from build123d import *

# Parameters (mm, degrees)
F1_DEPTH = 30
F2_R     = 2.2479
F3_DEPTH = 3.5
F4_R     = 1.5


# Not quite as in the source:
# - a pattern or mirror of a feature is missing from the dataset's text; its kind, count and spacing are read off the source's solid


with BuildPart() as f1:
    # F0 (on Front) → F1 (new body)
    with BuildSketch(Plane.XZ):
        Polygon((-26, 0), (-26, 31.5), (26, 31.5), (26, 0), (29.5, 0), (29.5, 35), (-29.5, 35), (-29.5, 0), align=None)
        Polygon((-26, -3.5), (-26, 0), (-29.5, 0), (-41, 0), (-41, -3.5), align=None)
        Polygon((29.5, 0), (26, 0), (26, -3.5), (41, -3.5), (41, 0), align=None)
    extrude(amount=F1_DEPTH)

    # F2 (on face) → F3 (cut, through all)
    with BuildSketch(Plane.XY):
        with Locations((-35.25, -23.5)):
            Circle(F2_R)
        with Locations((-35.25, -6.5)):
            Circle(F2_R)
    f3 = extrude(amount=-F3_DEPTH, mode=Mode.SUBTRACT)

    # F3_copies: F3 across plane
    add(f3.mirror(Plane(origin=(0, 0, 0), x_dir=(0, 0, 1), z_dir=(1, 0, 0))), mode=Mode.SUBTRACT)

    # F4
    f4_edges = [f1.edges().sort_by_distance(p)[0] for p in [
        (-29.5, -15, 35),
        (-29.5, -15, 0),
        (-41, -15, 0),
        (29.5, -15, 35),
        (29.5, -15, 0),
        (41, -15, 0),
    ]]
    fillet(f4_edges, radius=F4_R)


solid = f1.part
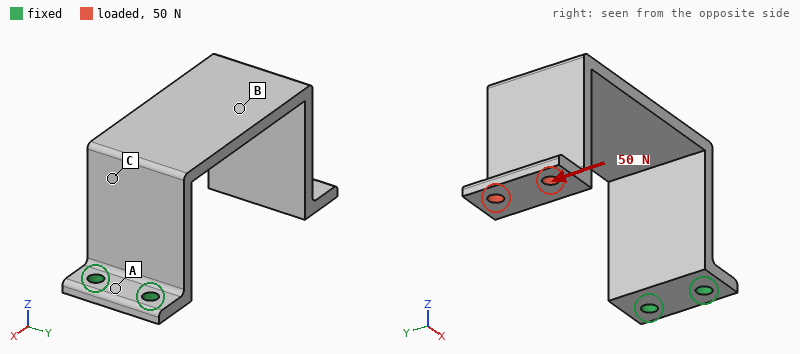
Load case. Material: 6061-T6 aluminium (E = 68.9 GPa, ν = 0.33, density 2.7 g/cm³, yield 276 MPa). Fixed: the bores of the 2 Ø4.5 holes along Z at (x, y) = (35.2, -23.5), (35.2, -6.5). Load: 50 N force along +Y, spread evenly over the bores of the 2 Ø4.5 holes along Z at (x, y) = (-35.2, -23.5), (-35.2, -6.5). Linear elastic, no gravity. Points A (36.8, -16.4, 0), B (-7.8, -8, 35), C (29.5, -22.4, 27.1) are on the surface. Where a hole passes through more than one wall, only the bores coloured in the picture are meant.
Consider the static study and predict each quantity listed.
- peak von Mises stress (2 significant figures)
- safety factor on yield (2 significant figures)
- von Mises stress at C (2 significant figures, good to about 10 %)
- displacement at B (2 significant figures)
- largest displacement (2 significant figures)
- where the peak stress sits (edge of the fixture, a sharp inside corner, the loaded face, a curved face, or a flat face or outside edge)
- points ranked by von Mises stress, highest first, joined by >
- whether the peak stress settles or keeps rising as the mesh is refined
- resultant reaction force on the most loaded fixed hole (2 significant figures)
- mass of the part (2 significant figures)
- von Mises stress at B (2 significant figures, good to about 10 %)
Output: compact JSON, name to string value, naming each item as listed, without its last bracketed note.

{"peak von Mises stress": "59 MPa", "safety factor on yield": "4.7", "von Mises stress at C": "40 MPa", "displacement at B": "0.29 mm", "largest displacement": "0.95 mm", "where the peak stress sits": "a curved face", "points ranked by von Mises stress, highest first, joined by >": "C > B > A", "whether the peak stress settles or keeps rising as the mesh is refined": "settles", "resultant reaction force on the most loaded fixed hole": "180 N", "mass of the part": "42 g", "von Mises stress at B": "24 MPa"}
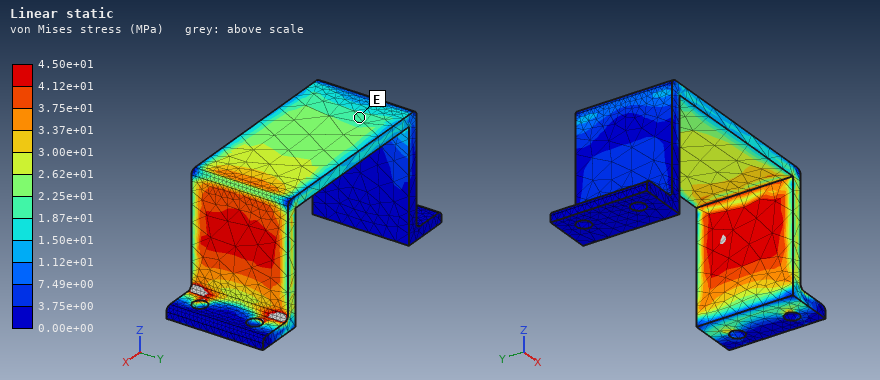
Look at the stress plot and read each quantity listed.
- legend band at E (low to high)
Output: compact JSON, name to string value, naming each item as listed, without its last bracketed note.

{"legend band at E": "1.87e+01 to 2.25e+01 MPa"}
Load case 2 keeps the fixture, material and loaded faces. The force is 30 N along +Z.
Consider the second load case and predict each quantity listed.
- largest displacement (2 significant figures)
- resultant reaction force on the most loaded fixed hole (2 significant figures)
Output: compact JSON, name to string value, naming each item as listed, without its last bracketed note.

{"largest displacement": "1.1 mm", "resultant reaction force on the most loaded fixed hole": "25 N"}
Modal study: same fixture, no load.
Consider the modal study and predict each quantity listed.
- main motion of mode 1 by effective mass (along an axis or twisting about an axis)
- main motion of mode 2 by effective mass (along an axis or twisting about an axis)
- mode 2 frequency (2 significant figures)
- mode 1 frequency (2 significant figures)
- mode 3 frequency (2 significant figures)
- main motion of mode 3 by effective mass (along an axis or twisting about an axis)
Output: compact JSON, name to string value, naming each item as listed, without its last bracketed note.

{"main motion of mode 1 by effective mass": "along Z", "main motion of mode 2 by effective mass": "along Y", "mode 2 frequency": "360 Hz", "mode 1 frequency": "230 Hz", "mode 3 frequency": "610 Hz", "main motion of mode 3 by effective mass": "along X"}
